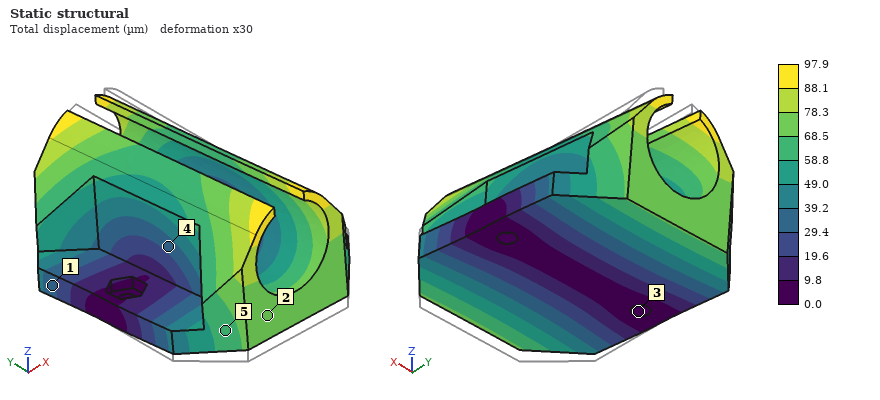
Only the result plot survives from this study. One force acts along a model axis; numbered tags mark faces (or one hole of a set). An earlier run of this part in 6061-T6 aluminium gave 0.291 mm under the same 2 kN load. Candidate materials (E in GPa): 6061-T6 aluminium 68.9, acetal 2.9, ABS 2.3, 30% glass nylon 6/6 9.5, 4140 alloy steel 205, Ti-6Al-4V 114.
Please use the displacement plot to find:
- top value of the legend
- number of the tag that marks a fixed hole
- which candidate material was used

97.9 µm
3
4140 alloy steel
